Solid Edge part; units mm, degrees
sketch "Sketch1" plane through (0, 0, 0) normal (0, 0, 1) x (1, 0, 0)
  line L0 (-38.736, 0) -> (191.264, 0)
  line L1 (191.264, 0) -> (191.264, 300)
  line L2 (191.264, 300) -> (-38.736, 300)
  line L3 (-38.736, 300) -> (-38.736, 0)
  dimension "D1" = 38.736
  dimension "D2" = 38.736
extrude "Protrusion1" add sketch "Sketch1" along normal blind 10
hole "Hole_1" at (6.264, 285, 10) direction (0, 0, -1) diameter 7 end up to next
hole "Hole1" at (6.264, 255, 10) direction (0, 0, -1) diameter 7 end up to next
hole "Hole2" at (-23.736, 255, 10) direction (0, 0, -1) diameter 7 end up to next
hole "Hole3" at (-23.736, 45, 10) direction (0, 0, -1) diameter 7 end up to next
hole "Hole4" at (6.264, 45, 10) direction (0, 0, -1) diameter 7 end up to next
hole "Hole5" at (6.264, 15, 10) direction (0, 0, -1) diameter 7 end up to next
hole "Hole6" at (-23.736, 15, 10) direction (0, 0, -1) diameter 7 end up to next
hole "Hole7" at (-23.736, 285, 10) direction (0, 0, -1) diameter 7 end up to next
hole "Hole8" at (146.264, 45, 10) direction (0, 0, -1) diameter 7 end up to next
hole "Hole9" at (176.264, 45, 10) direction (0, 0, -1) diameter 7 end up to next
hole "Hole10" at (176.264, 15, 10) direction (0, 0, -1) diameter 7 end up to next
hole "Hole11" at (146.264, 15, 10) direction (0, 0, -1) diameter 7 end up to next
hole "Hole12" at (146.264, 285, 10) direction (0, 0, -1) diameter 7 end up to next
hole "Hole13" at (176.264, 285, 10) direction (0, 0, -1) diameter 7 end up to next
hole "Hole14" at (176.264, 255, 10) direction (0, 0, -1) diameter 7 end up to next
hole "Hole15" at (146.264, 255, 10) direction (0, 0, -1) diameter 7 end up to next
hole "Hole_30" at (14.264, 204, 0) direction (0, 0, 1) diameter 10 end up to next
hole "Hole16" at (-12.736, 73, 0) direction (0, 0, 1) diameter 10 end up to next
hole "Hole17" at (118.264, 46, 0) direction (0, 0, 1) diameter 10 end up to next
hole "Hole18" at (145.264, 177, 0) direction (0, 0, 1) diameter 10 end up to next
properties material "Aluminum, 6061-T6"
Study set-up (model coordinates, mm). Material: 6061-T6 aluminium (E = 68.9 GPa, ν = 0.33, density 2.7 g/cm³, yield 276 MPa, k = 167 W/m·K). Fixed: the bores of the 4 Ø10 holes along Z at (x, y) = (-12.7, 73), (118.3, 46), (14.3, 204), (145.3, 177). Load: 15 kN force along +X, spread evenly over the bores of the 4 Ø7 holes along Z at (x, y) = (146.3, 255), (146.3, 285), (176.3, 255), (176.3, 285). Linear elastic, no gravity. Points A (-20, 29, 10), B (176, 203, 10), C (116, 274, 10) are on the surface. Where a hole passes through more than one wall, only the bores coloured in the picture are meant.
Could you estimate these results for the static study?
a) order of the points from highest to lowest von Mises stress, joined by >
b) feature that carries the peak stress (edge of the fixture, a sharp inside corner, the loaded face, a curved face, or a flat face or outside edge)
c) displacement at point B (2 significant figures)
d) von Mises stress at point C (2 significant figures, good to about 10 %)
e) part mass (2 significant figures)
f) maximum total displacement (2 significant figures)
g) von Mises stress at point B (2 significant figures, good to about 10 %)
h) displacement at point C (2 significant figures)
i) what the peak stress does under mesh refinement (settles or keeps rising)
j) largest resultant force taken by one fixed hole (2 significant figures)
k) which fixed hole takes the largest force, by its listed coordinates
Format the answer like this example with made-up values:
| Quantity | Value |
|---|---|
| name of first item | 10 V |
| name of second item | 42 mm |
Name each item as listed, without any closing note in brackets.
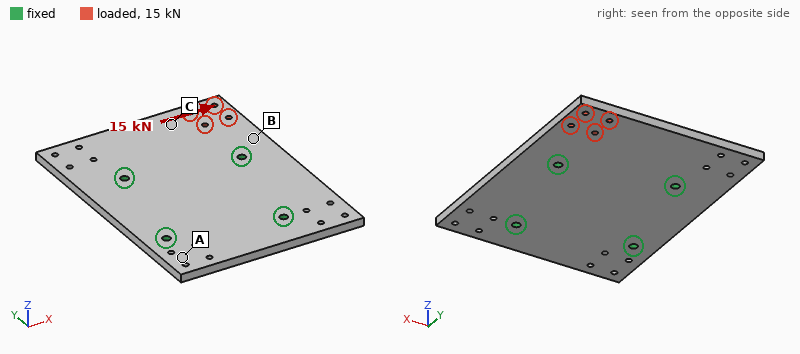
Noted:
| Quantity | Value |
|---|---|
| order of the points from highest to lowest von Mises stress, joined by > | C > B > A |
| feature that carries the peak stress | edge of the fixture |
| displacement at point B | 21 µm |
| von Mises stress at point C | 19 MPa |
| part mass | 1.8 kg |
| maximum total displacement | 69 µm |
| von Mises stress at point B | 10 MPa |
| displacement at point C | 42 µm |
| what the peak stress does under mesh refinement | keeps rising |
| largest resultant force taken by one fixed hole | 11 kN |
| which fixed hole takes the largest force, by its listed coordinates | (14.3, 204) |
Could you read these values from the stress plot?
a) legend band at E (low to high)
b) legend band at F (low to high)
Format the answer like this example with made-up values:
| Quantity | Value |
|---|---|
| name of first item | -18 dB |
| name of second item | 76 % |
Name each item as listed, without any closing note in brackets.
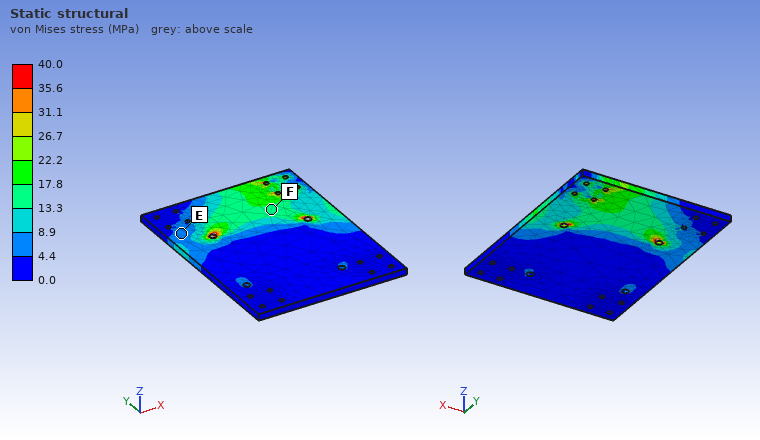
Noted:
| Quantity | Value |
|---|---|
| legend band at E | 4.4 to 8.9 MPa |
| legend band at F | 13.3 to 17.8 MPa |
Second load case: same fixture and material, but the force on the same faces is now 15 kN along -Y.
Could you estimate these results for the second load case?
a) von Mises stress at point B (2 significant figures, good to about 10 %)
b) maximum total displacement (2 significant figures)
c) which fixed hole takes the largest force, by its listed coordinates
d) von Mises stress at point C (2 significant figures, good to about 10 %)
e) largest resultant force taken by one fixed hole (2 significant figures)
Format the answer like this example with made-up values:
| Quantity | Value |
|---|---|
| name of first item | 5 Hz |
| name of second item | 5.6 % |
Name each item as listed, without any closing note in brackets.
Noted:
| Quantity | Value |
|---|---|
| von Mises stress at point B | 19 MPa |
| maximum total displacement | 50 µm |
| which fixed hole takes the largest force, by its listed coordinates | (145.3, 177) |
| von Mises stress at point C | 5.8 MPa |
| largest resultant force taken by one fixed hole | 12 kN |
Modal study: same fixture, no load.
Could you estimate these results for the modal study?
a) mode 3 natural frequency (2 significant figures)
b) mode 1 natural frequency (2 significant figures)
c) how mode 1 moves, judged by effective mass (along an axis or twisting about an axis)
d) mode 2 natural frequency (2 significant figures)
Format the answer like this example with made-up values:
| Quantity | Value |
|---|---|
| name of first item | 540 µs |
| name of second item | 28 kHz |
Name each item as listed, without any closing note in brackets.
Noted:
| Quantity | Value |
|---|---|
| mode 3 natural frequency | 1400 Hz |
| mode 1 natural frequency | 600 Hz |
| how mode 1 moves, judged by effective mass | along Z |
| mode 2 natural frequency | 1000 Hz |
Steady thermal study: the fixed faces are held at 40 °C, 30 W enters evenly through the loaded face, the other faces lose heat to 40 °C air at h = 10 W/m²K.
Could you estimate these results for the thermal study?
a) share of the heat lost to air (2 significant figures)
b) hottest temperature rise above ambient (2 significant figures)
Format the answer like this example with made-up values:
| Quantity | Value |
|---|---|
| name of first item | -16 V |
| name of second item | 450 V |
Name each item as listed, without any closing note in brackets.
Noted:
| Quantity | Value |
|---|---|
| share of the heat lost to air | 12 % |
| hottest temperature rise above ambient | 17 K |
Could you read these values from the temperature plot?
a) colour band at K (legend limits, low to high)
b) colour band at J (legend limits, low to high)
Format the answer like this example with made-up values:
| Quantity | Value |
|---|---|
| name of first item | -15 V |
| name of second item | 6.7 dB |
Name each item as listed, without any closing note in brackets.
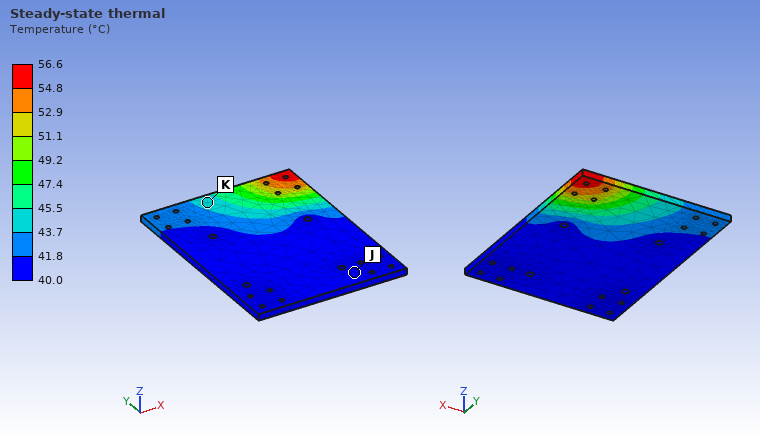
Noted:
| Quantity | Value |
|---|---|
| colour band at K | 43.7 to 45.5 °C |
| colour band at J | 40.0 to 41.8 °C |
